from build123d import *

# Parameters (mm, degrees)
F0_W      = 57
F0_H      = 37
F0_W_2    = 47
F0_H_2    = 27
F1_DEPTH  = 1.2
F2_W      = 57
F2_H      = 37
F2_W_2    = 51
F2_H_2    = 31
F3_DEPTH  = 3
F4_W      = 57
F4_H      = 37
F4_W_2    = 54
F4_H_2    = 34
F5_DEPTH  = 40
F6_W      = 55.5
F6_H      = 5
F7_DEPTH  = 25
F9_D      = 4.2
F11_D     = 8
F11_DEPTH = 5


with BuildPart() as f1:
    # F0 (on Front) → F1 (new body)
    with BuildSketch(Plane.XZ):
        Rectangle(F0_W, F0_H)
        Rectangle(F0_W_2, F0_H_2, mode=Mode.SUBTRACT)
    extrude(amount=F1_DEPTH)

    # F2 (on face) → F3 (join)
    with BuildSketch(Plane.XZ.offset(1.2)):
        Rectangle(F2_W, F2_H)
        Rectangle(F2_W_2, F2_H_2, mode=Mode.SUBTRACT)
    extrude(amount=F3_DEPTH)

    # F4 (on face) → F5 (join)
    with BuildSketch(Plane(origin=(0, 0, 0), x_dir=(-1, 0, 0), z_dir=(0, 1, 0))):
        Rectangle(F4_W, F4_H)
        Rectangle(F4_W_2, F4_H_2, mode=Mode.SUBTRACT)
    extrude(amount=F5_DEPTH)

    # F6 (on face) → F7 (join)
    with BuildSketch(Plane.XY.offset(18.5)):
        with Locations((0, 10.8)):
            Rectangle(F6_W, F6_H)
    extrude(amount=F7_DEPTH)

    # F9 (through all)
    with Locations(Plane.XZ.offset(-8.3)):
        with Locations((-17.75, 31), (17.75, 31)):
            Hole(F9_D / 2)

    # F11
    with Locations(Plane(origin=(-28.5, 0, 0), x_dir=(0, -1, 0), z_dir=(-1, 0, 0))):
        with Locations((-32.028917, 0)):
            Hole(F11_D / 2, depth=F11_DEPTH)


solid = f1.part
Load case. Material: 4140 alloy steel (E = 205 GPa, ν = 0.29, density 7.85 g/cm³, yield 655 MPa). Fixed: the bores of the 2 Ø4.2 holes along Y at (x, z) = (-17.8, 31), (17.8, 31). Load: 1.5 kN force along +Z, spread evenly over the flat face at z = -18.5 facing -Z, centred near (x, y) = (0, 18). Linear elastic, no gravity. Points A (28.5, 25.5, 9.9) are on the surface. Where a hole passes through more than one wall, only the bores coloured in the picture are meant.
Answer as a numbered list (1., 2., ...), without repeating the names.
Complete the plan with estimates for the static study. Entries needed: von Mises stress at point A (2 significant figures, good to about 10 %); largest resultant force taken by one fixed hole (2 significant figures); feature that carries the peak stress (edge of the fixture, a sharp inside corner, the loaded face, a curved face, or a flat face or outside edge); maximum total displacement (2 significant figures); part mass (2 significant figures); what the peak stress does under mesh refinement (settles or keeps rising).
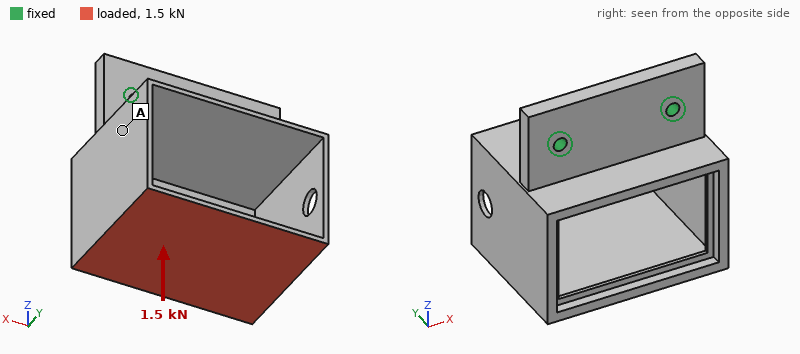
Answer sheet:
1. 46 MPa
2. 820 N
3. a sharp inside corner
4. 0.61 mm
5. 160 g
6. keeps rising
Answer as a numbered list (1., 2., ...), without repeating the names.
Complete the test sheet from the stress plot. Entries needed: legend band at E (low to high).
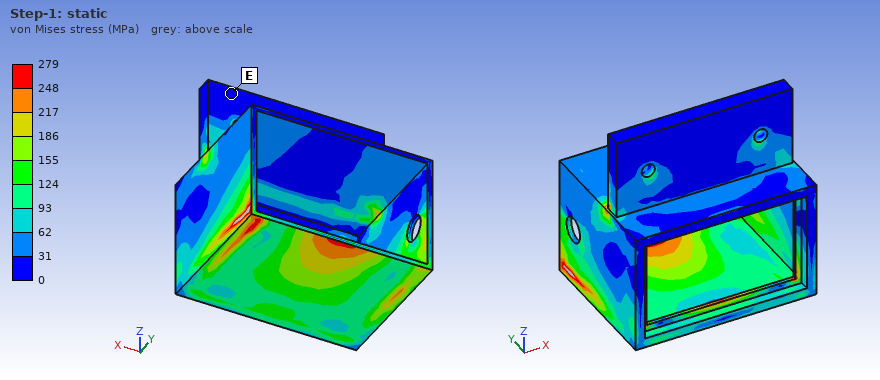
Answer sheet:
1. 0 to 31 MPa
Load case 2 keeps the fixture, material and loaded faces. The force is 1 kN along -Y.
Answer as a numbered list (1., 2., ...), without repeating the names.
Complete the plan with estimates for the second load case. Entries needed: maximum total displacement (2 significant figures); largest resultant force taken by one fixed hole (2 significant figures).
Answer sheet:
1. 0.73 mm
2. 500 N
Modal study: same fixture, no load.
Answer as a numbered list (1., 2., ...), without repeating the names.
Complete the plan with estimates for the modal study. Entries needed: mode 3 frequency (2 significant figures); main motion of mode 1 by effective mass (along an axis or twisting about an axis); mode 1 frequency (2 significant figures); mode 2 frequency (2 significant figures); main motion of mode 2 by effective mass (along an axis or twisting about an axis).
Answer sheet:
1. 1700 Hz
2. along Y
3. 870 Hz
4. 960 Hz
5. along X
